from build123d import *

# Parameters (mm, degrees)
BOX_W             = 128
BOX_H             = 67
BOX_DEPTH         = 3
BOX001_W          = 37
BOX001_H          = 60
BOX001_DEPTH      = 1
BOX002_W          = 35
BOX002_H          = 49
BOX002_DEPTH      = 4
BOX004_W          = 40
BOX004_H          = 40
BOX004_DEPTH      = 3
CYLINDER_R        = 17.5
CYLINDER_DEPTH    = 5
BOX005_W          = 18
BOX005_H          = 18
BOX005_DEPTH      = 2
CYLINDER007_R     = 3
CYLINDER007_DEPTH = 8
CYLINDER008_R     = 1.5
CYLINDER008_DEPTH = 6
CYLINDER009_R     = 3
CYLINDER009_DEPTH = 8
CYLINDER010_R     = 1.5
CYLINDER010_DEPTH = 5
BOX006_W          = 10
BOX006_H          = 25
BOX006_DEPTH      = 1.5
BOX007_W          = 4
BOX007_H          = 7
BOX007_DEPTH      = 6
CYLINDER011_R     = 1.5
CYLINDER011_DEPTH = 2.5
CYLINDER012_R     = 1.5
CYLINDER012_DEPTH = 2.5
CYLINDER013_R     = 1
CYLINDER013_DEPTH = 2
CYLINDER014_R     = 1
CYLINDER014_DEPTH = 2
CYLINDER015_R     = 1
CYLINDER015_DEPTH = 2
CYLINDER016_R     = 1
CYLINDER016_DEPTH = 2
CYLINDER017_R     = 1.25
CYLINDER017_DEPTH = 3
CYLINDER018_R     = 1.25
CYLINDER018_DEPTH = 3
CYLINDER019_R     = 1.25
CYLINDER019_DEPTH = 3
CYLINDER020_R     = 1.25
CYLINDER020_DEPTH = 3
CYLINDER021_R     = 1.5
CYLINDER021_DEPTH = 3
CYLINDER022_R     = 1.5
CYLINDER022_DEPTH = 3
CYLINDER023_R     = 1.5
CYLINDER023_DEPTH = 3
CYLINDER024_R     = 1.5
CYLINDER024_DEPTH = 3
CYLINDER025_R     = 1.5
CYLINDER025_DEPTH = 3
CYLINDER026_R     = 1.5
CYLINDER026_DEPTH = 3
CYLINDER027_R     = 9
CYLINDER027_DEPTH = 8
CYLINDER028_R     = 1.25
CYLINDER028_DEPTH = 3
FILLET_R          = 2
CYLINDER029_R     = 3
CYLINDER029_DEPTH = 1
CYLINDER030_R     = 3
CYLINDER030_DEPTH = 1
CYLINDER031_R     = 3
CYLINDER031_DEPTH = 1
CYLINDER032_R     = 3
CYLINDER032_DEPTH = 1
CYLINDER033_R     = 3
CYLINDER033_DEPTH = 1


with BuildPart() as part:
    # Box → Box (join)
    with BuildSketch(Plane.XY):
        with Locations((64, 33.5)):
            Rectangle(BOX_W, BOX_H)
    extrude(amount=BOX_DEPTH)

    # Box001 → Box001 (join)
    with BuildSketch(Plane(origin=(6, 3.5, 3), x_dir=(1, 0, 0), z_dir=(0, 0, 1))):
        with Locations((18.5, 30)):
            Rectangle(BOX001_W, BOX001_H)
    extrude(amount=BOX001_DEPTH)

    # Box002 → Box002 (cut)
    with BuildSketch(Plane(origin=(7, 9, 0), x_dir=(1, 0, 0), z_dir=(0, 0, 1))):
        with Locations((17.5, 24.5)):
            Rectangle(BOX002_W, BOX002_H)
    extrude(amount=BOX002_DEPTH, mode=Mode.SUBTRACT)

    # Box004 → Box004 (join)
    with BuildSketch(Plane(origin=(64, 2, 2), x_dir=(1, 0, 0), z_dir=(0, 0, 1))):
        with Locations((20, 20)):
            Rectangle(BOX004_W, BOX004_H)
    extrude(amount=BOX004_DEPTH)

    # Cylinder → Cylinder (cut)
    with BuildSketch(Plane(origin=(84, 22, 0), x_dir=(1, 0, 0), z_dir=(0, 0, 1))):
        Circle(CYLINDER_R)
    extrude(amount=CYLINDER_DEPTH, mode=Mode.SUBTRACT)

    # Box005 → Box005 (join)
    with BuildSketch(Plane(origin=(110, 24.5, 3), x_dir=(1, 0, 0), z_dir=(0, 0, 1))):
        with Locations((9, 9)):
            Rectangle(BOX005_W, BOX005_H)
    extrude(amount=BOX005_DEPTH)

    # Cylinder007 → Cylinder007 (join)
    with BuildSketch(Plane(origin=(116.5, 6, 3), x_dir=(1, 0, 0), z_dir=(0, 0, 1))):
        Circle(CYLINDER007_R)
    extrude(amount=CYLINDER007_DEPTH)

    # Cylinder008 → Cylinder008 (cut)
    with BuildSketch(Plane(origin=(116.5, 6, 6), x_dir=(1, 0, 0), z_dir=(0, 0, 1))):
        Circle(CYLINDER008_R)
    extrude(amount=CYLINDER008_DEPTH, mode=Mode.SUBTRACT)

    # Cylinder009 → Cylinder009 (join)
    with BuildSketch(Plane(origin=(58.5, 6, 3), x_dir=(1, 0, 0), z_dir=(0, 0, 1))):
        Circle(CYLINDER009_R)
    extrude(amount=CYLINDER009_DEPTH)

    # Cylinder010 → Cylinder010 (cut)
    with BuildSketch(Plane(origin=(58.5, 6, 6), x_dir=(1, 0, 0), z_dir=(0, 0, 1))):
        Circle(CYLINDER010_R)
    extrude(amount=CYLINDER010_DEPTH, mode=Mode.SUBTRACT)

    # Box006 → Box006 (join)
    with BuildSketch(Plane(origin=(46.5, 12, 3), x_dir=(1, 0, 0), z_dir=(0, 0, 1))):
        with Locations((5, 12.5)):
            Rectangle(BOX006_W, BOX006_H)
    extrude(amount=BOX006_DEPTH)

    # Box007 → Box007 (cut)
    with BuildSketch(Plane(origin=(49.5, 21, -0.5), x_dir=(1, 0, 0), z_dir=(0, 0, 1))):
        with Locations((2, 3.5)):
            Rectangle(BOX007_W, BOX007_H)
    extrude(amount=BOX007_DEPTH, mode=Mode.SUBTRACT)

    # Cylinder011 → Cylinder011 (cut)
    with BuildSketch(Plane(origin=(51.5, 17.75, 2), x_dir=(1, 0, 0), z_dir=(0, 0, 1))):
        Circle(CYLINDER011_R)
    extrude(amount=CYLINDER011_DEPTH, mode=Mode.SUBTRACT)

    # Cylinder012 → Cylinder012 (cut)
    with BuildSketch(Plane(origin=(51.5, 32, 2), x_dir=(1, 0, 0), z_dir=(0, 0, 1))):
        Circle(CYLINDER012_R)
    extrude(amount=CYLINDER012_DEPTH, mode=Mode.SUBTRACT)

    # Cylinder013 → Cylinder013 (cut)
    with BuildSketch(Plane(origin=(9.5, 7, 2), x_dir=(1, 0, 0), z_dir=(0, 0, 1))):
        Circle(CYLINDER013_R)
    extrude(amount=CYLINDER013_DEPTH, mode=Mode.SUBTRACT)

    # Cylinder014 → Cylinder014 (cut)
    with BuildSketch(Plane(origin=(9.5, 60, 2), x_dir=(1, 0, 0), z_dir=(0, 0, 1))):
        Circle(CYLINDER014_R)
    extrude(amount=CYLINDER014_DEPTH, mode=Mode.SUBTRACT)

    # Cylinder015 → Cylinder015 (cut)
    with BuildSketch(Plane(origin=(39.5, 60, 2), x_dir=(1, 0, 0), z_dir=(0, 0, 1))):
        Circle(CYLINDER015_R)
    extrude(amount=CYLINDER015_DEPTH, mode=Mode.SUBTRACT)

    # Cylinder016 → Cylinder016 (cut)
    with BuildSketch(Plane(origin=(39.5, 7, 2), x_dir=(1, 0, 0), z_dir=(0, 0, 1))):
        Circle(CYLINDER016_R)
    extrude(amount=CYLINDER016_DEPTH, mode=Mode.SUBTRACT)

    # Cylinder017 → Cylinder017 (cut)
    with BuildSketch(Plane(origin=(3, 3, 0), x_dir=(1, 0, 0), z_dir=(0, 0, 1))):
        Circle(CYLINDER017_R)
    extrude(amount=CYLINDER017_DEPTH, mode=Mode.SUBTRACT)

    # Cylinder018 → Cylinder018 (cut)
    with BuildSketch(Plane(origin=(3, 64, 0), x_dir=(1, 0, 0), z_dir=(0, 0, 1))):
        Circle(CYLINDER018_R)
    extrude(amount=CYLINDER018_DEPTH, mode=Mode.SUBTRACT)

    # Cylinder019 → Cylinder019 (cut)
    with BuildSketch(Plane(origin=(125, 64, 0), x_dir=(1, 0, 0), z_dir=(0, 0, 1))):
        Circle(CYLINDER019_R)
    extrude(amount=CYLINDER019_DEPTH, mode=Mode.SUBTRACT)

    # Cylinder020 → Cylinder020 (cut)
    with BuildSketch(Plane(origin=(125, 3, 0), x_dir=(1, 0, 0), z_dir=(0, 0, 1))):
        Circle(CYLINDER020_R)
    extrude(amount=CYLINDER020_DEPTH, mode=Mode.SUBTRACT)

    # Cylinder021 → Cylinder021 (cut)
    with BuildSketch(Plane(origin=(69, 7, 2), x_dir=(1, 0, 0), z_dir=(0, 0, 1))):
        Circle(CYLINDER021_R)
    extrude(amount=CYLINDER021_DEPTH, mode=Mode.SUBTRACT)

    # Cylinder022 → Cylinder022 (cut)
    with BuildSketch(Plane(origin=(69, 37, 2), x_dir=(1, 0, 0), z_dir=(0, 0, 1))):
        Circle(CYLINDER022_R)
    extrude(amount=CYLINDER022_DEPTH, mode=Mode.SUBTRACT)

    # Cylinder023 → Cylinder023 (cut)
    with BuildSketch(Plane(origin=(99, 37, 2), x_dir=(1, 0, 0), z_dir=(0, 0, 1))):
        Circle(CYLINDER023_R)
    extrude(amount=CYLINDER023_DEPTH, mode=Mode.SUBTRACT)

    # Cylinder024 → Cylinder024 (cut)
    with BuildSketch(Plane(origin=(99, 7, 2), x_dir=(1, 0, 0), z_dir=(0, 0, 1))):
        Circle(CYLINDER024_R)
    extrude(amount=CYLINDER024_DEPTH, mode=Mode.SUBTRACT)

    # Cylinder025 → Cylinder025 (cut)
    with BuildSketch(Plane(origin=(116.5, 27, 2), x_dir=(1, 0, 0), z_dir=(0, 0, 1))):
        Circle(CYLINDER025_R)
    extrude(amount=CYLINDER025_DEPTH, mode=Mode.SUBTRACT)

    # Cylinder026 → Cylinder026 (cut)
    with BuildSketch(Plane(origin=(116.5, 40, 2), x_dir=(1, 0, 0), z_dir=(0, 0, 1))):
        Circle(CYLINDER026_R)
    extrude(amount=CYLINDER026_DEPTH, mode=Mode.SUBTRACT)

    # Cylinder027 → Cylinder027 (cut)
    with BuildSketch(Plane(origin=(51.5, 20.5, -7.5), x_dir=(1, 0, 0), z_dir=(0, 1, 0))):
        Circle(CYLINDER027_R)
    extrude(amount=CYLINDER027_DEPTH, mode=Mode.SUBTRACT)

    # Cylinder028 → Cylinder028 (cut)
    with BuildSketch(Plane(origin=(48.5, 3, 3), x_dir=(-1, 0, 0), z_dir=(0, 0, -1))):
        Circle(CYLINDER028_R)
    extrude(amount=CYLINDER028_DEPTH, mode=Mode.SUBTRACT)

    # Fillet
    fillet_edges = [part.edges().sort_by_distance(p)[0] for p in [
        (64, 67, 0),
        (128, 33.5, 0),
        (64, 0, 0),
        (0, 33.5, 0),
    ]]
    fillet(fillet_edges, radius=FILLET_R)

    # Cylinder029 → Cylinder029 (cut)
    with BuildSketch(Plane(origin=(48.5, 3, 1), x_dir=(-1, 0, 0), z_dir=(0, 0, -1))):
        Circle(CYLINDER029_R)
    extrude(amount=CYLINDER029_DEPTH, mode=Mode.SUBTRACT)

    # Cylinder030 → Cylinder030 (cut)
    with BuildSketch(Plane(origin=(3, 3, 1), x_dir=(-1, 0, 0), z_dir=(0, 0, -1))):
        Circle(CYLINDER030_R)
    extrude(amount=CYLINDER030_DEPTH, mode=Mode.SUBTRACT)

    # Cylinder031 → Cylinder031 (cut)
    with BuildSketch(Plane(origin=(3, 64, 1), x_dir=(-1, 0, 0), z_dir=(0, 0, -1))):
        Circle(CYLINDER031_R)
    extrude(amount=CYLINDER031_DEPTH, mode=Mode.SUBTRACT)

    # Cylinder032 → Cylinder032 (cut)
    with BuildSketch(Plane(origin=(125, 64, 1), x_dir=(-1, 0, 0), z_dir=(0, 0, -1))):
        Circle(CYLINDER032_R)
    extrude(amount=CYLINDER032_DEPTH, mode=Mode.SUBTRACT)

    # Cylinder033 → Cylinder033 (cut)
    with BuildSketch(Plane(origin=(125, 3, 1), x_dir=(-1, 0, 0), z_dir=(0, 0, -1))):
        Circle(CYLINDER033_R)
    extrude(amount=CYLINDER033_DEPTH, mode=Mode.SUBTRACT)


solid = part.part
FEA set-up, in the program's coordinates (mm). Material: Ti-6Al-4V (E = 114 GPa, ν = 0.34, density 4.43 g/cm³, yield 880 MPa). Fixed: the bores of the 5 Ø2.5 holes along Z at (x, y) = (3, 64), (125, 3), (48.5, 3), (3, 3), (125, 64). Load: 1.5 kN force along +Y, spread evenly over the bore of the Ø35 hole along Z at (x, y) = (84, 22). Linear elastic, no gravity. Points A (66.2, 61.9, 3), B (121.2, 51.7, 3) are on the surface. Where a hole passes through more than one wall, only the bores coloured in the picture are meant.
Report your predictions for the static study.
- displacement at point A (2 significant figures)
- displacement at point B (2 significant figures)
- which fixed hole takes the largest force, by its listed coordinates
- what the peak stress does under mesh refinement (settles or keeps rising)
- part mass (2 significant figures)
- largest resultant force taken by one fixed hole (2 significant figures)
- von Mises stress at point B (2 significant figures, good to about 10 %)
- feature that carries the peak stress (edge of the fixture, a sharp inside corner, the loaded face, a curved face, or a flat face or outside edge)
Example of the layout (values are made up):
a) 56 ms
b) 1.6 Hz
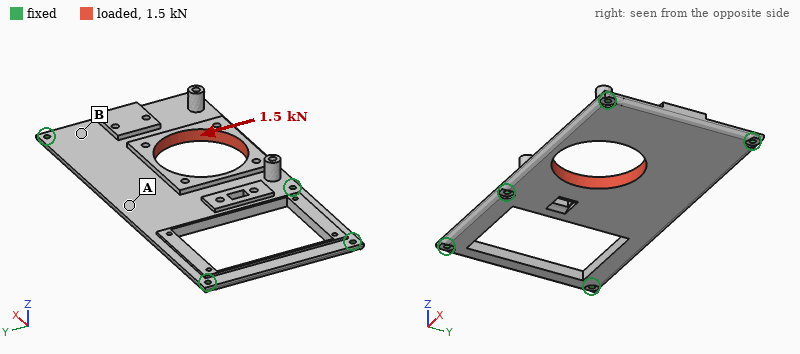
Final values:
a) 19 µm
b) 3.9 µm
c) (48.5, 3)
d) keeps rising
e) 89 g
f) 710 N
g) 14 MPa
h) edge of the fixture
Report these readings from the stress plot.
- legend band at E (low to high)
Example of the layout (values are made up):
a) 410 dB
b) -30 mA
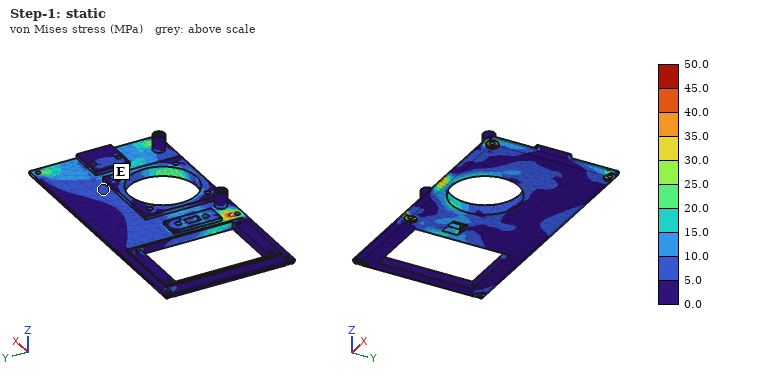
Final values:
a) 5.0 to 10.0 MPa
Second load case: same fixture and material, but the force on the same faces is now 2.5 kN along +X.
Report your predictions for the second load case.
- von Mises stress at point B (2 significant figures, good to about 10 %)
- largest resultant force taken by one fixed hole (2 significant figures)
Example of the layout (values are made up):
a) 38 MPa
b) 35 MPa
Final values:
a) 14 MPa
b) 790 N
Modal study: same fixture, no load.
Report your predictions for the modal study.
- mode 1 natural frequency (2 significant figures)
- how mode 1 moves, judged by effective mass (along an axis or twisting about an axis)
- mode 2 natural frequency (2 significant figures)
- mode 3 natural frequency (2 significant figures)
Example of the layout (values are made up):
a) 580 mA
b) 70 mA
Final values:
a) 1000 Hz
b) along Z
c) 2300 Hz
d) 3200 Hz
